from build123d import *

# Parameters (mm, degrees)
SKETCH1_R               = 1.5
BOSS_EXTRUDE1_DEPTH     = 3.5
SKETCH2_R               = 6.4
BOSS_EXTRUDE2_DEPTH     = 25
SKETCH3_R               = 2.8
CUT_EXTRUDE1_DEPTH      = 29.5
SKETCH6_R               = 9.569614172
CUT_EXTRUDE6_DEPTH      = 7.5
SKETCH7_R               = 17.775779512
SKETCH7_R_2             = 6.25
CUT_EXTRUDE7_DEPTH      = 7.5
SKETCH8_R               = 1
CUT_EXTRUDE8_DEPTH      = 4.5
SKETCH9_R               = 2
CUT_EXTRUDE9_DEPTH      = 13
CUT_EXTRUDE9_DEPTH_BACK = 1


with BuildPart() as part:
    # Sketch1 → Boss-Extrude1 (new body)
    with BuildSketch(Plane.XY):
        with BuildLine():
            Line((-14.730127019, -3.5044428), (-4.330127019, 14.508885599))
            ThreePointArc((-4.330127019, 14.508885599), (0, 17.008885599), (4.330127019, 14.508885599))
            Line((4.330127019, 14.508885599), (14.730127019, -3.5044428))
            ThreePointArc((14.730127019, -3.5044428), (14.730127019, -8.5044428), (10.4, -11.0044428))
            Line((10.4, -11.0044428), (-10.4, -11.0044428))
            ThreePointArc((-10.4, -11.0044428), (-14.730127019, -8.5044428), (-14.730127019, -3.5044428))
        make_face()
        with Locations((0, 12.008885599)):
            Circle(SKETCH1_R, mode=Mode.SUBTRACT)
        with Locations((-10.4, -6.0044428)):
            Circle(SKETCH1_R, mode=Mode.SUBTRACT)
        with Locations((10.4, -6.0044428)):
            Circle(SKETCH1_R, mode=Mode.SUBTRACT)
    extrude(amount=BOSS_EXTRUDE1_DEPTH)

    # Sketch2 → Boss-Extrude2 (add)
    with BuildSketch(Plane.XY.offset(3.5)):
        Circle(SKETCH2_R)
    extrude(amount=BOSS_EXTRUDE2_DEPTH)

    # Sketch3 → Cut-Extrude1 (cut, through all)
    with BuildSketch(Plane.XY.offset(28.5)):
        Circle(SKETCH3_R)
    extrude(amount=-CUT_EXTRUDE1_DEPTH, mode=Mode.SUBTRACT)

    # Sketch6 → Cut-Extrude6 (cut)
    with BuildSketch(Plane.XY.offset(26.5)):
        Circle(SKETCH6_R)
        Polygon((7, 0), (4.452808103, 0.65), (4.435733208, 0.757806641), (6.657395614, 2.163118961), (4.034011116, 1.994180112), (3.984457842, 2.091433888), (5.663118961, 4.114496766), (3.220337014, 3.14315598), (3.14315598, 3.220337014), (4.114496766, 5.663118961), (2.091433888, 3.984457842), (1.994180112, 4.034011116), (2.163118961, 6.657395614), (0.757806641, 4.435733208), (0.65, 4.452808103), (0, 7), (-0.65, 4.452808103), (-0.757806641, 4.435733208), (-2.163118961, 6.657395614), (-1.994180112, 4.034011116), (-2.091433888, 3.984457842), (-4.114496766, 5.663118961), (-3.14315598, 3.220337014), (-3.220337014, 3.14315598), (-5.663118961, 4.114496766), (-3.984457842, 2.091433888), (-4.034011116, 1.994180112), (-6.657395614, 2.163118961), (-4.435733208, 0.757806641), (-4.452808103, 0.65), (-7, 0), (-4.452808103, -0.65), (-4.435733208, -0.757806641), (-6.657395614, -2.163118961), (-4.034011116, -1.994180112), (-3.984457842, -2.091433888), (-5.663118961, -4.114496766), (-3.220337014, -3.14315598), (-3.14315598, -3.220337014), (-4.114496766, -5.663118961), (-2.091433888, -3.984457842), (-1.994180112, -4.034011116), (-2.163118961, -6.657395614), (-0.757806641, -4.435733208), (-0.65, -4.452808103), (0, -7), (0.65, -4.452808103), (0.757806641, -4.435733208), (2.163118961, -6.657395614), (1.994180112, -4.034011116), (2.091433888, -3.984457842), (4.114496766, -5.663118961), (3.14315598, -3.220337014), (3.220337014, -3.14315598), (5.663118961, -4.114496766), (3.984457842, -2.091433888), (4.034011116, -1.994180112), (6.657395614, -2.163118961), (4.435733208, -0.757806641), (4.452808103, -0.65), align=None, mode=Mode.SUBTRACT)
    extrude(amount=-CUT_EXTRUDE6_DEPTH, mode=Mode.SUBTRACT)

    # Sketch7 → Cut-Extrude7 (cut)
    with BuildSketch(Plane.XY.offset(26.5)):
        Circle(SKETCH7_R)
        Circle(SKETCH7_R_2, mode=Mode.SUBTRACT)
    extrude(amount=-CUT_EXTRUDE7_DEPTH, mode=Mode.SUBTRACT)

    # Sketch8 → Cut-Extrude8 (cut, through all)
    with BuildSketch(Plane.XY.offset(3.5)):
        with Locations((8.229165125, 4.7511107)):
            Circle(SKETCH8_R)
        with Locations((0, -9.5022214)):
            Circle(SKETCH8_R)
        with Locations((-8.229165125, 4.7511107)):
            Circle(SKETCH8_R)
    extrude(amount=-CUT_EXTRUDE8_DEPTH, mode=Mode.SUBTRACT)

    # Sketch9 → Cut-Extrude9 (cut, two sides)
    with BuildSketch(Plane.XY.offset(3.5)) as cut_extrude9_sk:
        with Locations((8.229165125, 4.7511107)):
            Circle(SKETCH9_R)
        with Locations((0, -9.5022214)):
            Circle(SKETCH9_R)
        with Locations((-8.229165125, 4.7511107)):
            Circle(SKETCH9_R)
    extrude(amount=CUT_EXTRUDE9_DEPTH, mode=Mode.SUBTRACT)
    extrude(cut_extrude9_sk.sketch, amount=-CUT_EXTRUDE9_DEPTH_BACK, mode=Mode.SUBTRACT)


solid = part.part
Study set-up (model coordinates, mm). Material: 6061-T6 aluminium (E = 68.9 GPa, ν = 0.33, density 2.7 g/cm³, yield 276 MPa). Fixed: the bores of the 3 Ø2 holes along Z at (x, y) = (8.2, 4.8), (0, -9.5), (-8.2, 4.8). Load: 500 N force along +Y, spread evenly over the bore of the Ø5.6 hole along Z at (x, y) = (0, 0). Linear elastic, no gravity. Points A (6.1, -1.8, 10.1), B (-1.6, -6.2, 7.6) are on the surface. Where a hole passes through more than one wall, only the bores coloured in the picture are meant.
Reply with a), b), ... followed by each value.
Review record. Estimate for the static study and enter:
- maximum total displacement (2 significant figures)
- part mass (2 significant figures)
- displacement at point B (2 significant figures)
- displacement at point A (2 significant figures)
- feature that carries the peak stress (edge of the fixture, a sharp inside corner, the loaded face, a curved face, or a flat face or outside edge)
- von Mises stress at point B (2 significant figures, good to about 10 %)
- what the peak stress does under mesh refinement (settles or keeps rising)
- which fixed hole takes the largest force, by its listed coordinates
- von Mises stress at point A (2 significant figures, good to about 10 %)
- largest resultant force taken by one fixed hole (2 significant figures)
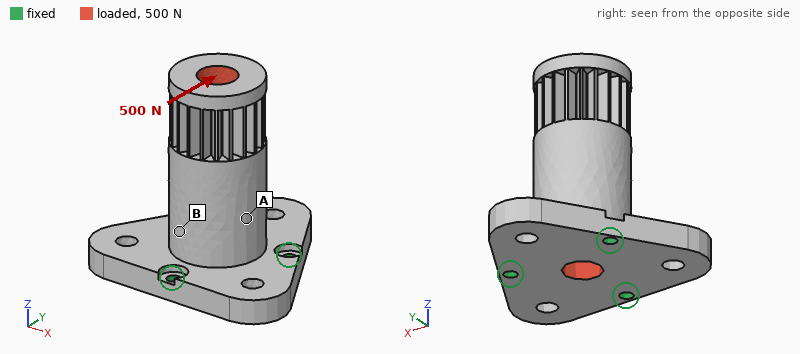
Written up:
a) 36 µm
b) 11 g
c) 8.9 µm
d) 9.5 µm
e) edge of the fixture
f) 22 MPa
g) keeps rising
h) (0, -9.5)
i) 8.0 MPa
j) 540 N
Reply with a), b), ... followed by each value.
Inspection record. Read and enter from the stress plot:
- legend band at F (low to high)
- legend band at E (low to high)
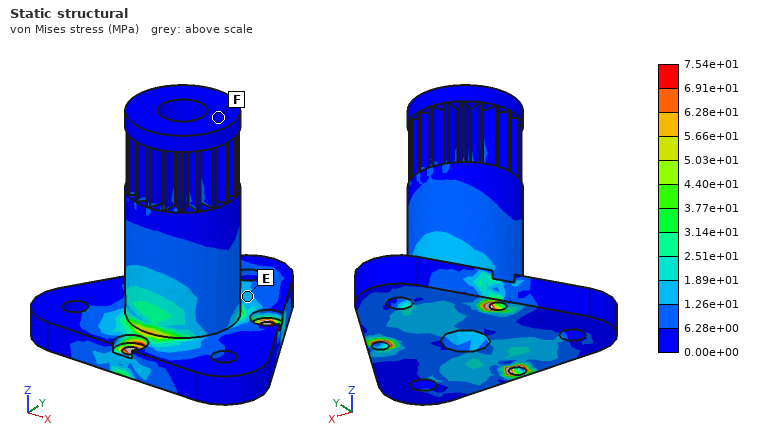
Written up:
a) 0.00e+00 to 6.28e+00 MPa
b) 1.26e+01 to 1.89e+01 MPa
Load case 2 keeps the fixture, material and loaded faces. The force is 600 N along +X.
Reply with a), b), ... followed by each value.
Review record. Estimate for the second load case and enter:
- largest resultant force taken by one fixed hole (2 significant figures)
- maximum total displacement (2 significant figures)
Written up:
a) 560 N
b) 43 µm
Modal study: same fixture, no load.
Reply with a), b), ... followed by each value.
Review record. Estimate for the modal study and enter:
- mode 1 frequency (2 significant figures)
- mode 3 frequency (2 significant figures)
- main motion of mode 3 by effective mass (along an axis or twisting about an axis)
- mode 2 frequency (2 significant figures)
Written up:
a) 8700 Hz
b) 20 kHz
c) along Z
d) 8700 Hz
